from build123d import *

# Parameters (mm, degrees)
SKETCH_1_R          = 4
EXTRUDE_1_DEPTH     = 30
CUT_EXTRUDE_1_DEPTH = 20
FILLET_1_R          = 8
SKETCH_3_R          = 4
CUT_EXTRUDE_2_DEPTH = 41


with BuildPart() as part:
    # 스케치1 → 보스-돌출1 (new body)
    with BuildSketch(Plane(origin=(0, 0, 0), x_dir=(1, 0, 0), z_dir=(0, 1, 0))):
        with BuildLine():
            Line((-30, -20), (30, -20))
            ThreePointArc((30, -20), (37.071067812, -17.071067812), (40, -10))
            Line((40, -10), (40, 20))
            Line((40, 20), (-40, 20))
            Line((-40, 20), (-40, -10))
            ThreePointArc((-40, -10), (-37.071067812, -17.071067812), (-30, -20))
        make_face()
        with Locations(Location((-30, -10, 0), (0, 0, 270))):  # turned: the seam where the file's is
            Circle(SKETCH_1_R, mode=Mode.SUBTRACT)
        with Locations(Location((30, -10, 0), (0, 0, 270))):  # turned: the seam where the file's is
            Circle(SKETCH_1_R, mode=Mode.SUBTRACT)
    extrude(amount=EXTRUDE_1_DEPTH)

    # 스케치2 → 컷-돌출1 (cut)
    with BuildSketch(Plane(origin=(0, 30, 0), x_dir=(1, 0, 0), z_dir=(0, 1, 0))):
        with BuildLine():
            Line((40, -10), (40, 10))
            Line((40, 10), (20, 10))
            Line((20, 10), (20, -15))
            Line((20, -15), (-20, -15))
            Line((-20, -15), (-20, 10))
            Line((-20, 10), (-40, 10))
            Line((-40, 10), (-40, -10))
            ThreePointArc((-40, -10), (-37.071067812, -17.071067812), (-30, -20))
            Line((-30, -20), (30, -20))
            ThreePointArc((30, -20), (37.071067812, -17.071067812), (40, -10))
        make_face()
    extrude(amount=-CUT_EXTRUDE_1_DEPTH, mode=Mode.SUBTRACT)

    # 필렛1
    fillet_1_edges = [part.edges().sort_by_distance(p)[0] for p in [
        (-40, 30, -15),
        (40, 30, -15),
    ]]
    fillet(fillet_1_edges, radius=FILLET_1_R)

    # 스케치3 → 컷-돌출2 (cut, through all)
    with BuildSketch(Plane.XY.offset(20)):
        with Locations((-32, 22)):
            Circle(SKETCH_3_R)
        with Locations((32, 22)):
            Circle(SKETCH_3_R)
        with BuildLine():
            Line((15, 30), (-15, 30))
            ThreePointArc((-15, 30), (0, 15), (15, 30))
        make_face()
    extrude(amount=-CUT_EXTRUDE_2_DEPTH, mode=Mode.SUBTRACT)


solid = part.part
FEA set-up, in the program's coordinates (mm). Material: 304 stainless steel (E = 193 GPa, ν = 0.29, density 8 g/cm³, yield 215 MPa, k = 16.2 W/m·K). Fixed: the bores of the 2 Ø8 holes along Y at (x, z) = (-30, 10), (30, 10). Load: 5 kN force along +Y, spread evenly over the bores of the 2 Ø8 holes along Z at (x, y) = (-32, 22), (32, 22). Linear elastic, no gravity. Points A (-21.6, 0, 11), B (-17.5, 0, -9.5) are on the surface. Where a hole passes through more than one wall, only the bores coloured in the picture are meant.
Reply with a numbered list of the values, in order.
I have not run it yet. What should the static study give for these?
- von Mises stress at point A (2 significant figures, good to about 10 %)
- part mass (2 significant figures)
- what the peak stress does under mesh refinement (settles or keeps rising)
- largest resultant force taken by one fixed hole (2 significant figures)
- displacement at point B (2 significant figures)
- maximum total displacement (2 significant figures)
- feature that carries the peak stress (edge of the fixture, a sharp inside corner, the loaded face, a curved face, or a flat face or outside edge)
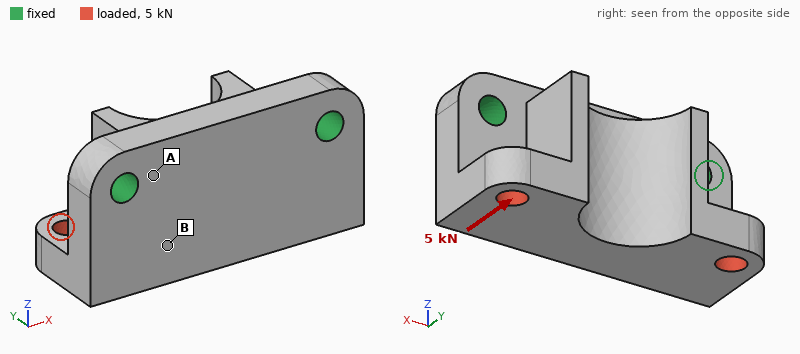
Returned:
1. 52 MPa
2. 420 g
3. keeps rising
4. 2.5 kN
5. 18 µm
6. 39 µm
7. edge of the fixture
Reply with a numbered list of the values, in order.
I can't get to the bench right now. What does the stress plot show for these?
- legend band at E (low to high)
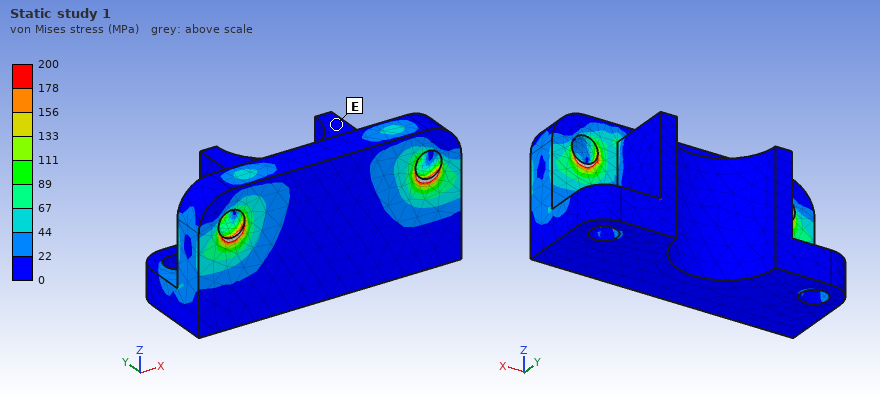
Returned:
1. 0 to 22 MPa
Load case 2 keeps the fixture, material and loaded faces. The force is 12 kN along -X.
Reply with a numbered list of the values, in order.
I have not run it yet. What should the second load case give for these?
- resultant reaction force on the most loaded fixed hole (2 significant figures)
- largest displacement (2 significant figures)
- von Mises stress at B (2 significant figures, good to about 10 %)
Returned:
1. 8.3 kN
2. 25 µm
3. 12 MPa
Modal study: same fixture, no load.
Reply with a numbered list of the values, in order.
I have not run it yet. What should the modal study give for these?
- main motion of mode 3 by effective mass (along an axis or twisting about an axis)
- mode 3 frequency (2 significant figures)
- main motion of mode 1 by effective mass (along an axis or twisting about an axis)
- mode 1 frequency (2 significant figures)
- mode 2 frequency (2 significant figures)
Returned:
1. along Y
2. 11 kHz
3. along Y
4. 4400 Hz
5. 8800 Hz
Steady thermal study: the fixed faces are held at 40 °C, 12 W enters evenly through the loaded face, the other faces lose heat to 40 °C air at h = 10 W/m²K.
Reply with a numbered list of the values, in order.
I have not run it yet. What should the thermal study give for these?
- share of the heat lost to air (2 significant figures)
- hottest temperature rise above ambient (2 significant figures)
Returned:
1. 17 %
2. 46 K
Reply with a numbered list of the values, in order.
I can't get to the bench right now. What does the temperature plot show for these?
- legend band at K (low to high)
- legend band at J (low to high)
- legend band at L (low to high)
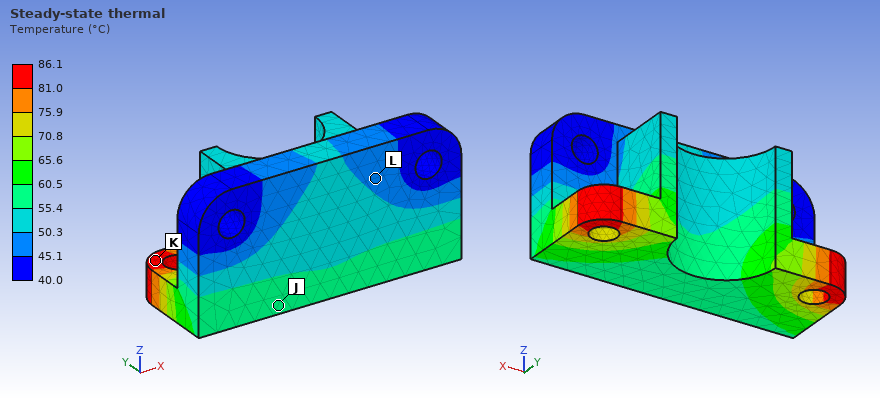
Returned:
1. 81.0 to 86.1 °C
2. 55.4 to 60.5 °C
3. 45.1 to 50.3 °C
